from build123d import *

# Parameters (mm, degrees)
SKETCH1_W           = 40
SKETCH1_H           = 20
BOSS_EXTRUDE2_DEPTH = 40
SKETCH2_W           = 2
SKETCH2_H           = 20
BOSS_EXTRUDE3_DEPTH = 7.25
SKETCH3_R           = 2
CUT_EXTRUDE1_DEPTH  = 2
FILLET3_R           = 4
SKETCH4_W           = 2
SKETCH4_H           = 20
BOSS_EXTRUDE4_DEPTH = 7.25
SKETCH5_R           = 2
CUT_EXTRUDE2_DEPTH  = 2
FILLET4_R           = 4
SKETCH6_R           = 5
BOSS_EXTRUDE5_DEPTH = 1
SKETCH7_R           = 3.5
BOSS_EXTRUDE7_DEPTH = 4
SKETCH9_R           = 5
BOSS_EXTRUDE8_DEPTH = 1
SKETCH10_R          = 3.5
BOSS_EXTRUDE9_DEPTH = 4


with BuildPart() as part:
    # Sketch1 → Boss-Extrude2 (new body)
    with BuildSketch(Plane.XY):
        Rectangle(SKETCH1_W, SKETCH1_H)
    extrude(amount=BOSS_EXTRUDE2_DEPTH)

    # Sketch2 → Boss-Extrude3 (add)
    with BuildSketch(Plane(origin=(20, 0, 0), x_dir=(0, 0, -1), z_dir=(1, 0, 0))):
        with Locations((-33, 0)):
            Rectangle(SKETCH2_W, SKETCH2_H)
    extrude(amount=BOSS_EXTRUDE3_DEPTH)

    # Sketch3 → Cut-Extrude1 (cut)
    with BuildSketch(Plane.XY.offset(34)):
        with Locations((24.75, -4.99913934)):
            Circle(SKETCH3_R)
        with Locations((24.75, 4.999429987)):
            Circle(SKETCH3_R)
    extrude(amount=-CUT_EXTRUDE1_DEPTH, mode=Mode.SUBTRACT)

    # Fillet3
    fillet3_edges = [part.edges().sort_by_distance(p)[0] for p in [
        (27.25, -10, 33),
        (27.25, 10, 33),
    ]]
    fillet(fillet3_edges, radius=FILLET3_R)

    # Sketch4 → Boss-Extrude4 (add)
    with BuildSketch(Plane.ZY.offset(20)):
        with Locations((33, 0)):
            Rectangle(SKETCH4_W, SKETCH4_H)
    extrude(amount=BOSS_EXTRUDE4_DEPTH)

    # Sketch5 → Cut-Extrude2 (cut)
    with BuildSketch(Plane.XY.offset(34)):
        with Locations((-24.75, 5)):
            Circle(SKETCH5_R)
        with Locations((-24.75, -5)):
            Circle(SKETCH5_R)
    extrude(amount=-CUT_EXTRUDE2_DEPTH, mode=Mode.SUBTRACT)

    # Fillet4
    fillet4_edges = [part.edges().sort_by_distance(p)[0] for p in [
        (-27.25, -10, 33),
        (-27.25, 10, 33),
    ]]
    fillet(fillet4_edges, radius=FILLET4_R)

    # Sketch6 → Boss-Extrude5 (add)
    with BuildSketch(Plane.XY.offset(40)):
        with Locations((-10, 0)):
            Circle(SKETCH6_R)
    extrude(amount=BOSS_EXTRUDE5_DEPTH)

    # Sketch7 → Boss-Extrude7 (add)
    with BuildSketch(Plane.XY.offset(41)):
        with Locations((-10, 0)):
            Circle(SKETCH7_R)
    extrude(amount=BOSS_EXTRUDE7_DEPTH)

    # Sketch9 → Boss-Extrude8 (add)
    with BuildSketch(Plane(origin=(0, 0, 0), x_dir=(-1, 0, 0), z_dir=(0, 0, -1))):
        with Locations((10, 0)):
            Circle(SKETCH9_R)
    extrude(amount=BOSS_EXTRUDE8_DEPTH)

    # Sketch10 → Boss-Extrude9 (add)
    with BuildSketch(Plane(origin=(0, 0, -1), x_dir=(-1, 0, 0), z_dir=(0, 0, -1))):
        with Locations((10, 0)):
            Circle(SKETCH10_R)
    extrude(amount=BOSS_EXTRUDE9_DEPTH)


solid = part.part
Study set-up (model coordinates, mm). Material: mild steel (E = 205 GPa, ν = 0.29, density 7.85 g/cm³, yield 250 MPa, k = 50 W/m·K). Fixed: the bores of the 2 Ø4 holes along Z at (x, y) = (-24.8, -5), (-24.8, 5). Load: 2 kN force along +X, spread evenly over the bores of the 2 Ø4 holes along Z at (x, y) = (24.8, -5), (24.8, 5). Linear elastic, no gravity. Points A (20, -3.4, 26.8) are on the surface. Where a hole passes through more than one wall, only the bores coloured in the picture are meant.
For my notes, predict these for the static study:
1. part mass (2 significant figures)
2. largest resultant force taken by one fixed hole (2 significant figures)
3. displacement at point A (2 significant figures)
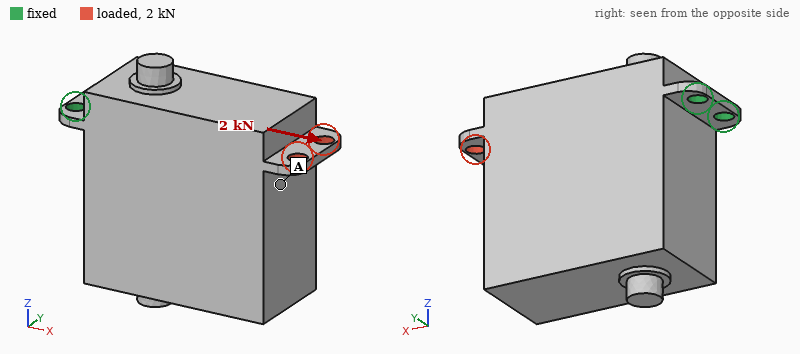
260 g
1.0 kN
2.4 µm
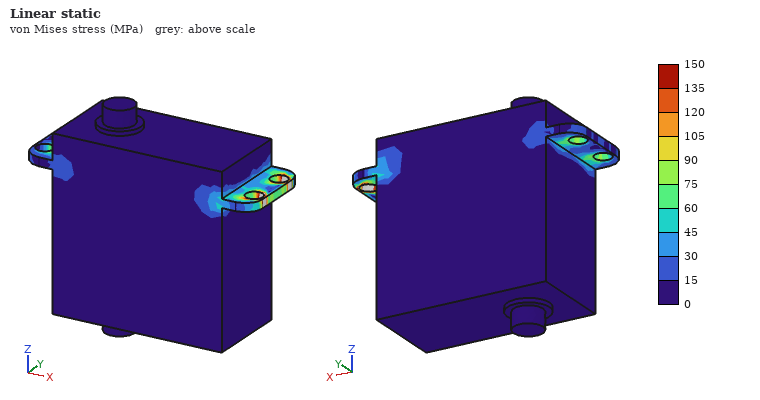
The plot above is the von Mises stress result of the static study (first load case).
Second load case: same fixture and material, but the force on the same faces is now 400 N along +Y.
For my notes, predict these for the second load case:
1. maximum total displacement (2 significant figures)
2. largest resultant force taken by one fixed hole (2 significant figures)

32 µm
1.6 kN
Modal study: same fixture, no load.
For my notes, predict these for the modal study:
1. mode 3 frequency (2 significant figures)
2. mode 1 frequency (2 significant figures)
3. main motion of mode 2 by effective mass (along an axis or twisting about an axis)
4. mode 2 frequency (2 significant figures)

3000 Hz
280 Hz
along Y
1400 Hz
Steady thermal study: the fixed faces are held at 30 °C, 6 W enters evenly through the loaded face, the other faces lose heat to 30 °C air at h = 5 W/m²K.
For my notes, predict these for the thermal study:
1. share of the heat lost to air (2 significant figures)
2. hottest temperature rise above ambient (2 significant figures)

11 %
53 K
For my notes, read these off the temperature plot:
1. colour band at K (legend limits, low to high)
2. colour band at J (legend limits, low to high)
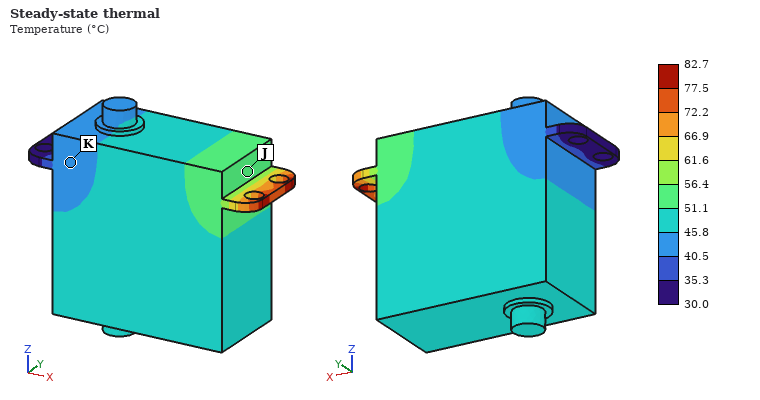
40.5 to 45.8 °C
51.1 to 56.4 °C
